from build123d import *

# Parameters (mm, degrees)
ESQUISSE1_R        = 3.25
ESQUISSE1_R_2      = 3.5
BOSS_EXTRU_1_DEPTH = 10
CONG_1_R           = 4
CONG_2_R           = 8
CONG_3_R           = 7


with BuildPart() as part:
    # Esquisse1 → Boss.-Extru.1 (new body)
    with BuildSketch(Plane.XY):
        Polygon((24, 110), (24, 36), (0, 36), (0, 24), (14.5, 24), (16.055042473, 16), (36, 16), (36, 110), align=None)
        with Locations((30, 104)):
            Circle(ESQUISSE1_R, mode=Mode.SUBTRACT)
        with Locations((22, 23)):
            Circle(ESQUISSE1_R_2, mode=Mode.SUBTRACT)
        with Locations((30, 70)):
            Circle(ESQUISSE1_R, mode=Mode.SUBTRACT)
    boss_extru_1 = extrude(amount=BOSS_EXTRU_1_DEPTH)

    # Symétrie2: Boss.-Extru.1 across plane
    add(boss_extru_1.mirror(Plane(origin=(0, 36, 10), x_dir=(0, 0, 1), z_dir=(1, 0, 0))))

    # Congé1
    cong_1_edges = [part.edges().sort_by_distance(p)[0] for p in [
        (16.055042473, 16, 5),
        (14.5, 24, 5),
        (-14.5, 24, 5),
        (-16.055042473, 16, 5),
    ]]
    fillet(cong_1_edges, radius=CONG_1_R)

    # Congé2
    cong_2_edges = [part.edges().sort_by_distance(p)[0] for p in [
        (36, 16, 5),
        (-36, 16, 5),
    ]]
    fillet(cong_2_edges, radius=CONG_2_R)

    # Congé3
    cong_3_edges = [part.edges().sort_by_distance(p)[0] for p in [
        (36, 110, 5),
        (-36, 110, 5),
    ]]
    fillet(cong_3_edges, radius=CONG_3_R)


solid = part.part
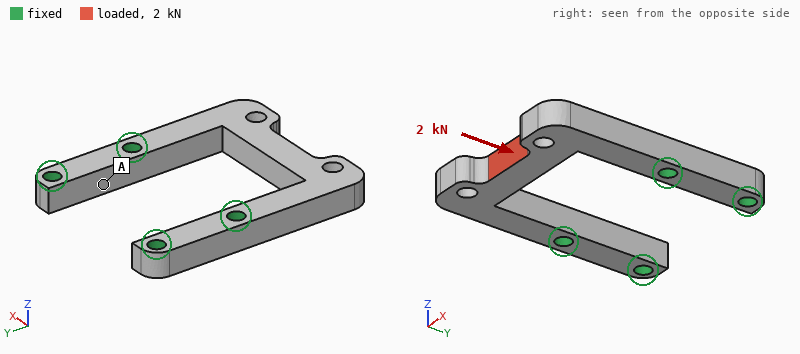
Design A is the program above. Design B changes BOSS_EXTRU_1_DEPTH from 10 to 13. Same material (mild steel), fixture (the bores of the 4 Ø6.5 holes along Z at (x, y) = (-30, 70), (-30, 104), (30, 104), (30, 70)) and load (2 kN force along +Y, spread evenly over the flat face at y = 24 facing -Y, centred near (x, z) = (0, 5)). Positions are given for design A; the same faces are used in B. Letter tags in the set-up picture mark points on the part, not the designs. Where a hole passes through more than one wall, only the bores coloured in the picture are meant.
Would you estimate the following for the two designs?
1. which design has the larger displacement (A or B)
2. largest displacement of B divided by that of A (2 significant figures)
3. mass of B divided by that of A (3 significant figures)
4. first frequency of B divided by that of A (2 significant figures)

A
0.77
1.30
1.3
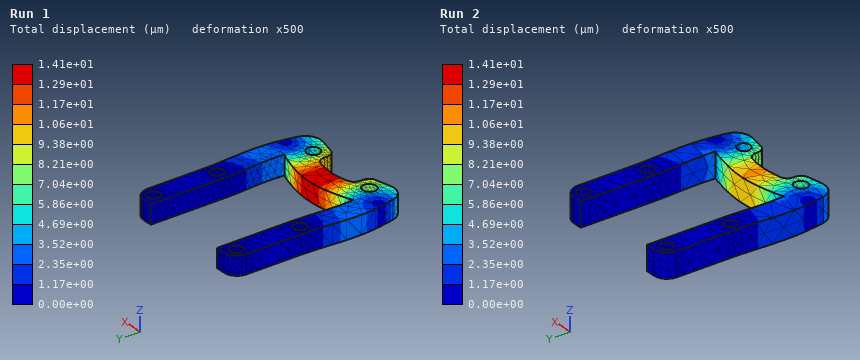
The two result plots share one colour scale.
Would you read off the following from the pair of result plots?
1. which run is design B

Run 2
